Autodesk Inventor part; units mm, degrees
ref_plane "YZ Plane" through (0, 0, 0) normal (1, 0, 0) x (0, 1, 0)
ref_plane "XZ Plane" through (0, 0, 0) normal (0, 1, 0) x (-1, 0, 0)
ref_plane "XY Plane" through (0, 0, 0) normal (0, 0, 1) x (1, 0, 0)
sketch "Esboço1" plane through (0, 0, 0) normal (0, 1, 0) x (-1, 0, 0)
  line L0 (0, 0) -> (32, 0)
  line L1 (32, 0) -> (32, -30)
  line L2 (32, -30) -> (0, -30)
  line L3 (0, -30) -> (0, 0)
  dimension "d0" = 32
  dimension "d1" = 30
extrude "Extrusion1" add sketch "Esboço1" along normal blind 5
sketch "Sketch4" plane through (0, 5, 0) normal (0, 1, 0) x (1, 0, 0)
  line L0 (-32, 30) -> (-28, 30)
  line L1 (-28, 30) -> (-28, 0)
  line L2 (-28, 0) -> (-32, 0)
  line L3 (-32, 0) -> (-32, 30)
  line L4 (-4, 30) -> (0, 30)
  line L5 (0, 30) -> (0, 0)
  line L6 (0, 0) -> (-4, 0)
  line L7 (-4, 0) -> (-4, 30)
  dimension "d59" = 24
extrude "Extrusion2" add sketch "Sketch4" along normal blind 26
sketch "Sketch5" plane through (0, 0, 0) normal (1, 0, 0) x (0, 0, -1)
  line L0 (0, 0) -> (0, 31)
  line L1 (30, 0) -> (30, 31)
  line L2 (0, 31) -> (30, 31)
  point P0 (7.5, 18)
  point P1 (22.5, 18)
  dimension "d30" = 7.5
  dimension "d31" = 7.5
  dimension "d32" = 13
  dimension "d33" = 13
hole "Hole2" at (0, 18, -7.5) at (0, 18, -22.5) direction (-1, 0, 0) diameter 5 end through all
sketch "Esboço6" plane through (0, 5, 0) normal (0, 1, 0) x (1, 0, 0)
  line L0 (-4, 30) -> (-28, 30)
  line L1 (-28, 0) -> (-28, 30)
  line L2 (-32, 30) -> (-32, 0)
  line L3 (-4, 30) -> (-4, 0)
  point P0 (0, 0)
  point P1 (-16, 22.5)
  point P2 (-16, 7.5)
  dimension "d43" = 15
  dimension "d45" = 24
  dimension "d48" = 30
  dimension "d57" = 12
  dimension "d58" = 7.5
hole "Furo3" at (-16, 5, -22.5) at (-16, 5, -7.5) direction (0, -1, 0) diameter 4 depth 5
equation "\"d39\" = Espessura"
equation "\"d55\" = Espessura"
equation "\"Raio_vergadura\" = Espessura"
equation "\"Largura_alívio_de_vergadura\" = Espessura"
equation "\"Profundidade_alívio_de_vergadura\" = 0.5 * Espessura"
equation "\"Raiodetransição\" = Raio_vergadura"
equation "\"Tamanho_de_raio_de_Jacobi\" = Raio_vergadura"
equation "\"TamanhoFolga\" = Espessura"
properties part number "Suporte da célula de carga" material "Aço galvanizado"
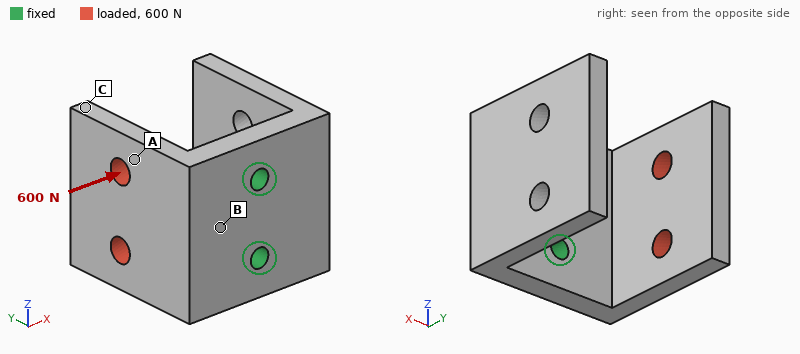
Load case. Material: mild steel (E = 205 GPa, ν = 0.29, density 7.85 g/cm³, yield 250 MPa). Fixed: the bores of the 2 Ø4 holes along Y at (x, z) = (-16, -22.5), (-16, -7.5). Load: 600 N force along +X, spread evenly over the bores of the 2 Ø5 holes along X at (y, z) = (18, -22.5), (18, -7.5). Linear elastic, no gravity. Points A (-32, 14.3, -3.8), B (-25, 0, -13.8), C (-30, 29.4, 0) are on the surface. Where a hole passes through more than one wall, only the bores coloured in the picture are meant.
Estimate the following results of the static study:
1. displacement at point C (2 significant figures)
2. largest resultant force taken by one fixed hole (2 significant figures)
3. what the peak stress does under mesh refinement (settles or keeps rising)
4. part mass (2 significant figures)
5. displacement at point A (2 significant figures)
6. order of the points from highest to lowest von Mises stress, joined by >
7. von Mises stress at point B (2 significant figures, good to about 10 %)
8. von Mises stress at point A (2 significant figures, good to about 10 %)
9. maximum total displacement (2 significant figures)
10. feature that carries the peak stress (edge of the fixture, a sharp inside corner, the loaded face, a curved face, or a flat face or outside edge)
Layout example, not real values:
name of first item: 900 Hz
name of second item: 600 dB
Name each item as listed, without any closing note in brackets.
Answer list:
displacement at point C: 89 µm
largest resultant force taken by one fixed hole: 310 N
what the peak stress does under mesh refinement: keeps rising
part mass: 83 g
displacement at point A: 39 µm
order of the points from highest to lowest von Mises stress, joined by >: B > A > C
von Mises stress at point B: 61 MPa
von Mises stress at point A: 33 MPa
maximum total displacement: 98 µm
feature that carries the peak stress: edge of the fixture
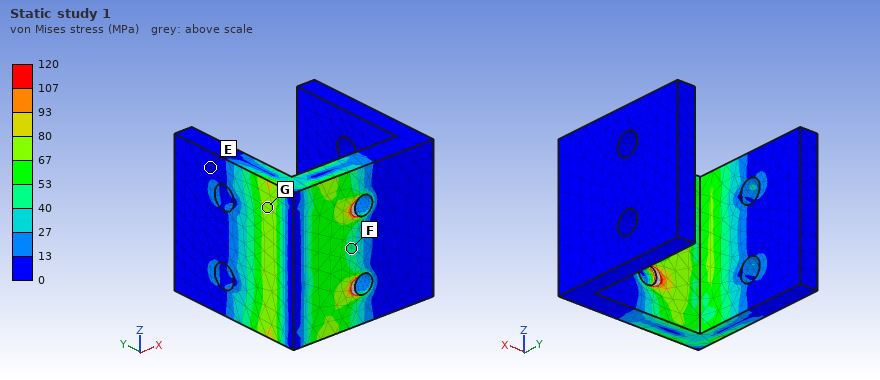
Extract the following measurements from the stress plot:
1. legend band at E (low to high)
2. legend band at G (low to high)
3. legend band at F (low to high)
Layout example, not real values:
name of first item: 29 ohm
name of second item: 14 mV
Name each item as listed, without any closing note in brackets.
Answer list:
legend band at E: 0 to 13 MPa
legend band at G: 67 to 80 MPa
legend band at F: 40 to 53 MPa
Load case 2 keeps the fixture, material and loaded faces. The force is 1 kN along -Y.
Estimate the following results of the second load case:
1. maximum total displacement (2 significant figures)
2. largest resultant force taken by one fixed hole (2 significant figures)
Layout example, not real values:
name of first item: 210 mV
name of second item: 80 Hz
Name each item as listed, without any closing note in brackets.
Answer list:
maximum total displacement: 46 µm
largest resultant force taken by one fixed hole: 500 N
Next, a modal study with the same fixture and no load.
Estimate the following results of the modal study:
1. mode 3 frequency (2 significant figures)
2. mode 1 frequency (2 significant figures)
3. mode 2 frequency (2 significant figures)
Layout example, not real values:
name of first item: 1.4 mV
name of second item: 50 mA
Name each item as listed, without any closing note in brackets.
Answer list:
mode 3 frequency: 5600 Hz
mode 1 frequency: 2900 Hz
mode 2 frequency: 3000 Hz
